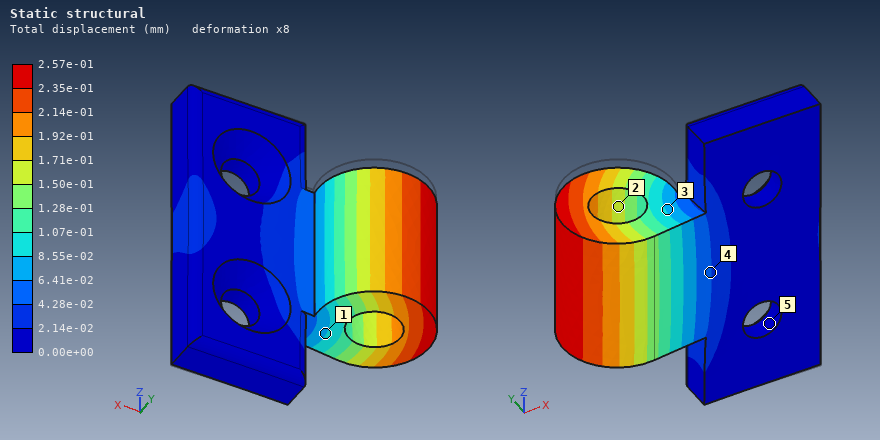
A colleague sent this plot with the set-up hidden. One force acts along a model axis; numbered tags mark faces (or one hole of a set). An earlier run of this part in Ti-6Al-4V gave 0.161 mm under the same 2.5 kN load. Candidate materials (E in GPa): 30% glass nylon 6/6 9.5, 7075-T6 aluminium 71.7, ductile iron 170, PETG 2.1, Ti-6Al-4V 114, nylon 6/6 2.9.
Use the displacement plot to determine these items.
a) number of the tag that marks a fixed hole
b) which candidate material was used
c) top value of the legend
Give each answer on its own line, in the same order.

5
7075-T6 aluminium
2.57e-01 mm
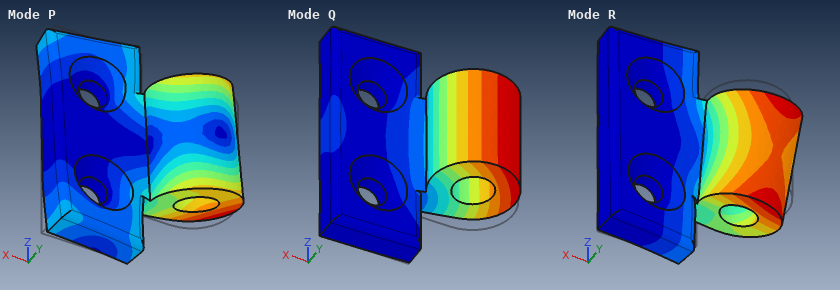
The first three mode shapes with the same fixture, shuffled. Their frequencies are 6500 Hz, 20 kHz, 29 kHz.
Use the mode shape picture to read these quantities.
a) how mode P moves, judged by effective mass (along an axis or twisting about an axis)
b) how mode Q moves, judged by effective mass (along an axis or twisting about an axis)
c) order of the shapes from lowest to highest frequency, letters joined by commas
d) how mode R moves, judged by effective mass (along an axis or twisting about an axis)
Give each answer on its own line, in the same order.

along Z
along Y
Q, R, P
along Z
